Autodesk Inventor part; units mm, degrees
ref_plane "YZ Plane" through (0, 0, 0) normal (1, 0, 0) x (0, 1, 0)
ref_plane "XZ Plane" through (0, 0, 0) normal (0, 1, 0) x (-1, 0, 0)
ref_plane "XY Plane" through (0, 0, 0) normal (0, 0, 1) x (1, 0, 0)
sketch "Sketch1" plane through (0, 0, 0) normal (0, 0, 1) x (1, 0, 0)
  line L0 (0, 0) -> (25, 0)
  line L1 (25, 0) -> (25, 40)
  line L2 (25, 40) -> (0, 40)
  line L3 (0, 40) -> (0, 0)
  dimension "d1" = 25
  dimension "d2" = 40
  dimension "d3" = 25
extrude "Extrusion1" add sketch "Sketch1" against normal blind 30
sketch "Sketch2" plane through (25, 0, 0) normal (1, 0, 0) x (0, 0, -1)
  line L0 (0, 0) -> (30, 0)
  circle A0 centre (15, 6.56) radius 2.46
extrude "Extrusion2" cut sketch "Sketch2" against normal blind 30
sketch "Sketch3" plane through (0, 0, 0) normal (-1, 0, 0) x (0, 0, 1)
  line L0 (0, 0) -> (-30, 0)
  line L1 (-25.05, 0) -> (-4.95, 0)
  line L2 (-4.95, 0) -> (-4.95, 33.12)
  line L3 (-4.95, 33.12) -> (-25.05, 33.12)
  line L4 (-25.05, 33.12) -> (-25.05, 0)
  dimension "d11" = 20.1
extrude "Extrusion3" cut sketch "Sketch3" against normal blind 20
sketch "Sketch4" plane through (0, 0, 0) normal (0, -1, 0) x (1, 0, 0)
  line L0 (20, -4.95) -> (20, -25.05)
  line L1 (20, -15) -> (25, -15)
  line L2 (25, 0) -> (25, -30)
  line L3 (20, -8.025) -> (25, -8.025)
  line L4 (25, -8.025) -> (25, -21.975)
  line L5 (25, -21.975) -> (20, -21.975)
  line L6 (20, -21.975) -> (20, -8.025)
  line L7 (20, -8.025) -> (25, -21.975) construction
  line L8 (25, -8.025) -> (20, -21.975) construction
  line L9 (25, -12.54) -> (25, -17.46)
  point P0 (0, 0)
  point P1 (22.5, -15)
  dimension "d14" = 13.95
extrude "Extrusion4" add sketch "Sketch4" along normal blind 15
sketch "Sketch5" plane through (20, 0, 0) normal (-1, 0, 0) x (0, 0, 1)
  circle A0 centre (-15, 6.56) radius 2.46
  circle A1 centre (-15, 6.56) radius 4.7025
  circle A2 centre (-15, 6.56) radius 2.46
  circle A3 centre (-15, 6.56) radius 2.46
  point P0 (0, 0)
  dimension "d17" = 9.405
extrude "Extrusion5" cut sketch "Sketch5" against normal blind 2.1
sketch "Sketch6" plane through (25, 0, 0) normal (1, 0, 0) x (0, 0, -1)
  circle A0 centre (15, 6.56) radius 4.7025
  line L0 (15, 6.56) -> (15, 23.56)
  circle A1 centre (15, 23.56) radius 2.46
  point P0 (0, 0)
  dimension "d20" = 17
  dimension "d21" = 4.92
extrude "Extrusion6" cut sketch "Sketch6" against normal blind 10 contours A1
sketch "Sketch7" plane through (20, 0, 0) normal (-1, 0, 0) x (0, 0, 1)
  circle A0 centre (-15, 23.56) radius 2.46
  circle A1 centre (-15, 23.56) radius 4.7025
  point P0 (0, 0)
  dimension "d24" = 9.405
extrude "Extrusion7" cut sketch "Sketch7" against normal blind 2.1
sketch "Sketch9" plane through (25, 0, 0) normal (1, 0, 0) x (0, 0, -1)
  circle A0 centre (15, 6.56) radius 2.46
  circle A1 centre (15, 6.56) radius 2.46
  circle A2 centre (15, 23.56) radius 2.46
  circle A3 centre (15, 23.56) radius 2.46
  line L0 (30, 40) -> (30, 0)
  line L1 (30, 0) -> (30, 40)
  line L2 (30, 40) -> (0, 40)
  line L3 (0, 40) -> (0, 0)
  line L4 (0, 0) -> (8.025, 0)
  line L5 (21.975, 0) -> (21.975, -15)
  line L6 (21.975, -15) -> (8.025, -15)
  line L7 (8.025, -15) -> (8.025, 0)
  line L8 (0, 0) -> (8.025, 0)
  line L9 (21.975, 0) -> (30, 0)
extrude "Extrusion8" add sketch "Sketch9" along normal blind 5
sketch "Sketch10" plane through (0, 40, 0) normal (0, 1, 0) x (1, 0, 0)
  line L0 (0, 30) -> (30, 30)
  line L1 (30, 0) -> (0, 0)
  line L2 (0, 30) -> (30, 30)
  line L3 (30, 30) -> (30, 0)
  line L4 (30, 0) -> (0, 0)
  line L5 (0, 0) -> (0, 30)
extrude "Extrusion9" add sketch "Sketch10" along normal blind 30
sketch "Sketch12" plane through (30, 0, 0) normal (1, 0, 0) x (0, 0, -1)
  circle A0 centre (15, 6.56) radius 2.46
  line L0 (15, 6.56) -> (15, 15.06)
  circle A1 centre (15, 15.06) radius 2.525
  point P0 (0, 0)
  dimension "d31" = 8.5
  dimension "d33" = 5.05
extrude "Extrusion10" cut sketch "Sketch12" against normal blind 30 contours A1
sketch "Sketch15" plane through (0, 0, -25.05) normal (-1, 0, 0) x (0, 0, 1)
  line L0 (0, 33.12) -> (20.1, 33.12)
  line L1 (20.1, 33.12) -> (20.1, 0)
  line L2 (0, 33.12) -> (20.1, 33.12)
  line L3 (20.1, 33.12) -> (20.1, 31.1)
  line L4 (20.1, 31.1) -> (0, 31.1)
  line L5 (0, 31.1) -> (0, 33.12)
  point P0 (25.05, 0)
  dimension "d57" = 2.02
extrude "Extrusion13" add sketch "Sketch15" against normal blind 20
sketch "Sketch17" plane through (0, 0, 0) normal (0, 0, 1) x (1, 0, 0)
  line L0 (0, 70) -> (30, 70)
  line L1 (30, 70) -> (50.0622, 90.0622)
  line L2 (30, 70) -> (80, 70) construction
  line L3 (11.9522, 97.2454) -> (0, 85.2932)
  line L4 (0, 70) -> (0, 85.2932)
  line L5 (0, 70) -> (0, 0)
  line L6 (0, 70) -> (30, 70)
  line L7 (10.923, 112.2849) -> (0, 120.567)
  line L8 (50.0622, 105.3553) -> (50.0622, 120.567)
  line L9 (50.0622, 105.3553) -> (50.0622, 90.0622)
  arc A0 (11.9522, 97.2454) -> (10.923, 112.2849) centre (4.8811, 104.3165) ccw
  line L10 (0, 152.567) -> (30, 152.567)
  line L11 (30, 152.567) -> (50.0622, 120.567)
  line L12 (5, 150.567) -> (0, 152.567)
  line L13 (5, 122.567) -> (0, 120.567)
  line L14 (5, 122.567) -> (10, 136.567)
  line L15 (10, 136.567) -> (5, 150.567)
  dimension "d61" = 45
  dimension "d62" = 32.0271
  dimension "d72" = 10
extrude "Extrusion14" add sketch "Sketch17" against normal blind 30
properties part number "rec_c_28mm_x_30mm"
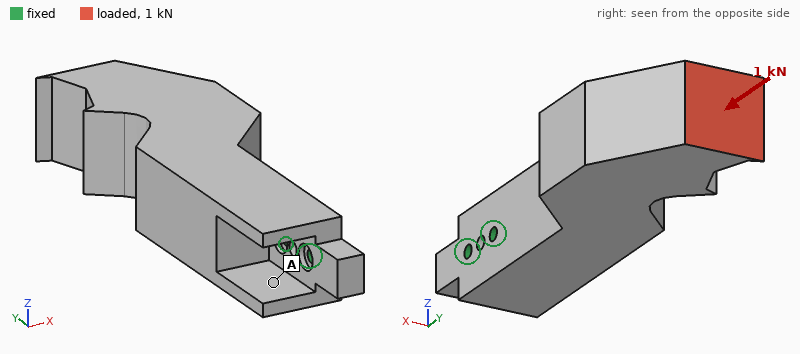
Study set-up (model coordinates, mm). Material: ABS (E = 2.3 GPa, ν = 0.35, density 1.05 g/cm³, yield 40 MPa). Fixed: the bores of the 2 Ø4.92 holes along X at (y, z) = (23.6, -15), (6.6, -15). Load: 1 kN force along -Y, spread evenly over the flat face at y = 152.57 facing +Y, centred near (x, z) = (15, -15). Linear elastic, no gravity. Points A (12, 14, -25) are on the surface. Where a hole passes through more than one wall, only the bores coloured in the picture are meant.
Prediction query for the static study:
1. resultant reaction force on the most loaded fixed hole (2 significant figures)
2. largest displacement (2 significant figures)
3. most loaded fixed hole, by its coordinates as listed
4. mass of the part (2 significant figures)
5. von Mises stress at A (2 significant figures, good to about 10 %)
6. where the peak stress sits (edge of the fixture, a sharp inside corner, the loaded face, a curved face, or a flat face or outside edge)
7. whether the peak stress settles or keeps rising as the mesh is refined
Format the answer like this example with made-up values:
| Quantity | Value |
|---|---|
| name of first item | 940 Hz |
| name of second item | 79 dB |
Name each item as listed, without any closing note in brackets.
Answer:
| Quantity | Value |
|---|---|
| resultant reaction force on the most loaded fixed hole | 750 N |
| largest displacement | 1.3 mm |
| most loaded fixed hole, by its coordinates as listed | (23.6, -15) |
| mass of the part | 150 g |
| von Mises stress at A | 3.4 MPa |
| where the peak stress sits | edge of the fixture |
| whether the peak stress settles or keeps rising as the mesh is refined | keeps rising |
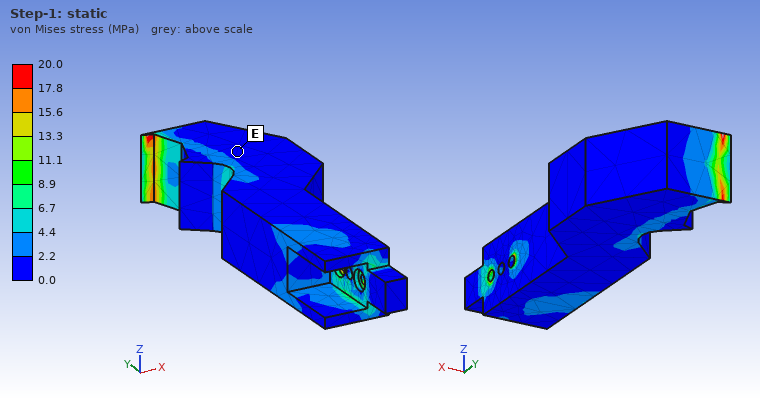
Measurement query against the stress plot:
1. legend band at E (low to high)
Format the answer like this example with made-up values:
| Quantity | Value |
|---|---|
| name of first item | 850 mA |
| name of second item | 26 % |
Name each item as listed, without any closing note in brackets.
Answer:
| Quantity | Value |
|---|---|
| legend band at E | 0.0 to 2.2 MPa |
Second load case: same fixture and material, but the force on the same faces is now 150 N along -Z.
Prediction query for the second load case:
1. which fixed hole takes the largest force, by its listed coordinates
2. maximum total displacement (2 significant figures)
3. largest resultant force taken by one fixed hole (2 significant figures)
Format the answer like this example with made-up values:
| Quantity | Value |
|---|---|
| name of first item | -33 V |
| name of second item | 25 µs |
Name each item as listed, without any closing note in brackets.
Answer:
| Quantity | Value |
|---|---|
| which fixed hole takes the largest force, by its listed coordinates | (23.6, -15) |
| maximum total displacement | 1.8 mm |
| largest resultant force taken by one fixed hole | 990 N |
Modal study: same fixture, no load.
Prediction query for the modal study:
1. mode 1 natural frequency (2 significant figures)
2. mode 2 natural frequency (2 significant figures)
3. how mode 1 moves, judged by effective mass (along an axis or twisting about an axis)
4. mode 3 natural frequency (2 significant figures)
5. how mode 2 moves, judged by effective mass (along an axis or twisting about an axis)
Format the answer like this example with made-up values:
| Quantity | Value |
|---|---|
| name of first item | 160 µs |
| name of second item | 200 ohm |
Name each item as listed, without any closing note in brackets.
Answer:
| Quantity | Value |
|---|---|
| mode 1 natural frequency | 190 Hz |
| mode 2 natural frequency | 220 Hz |
| how mode 1 moves, judged by effective mass | along X |
| mode 3 natural frequency | 670 Hz |
| how mode 2 moves, judged by effective mass | along Z |
